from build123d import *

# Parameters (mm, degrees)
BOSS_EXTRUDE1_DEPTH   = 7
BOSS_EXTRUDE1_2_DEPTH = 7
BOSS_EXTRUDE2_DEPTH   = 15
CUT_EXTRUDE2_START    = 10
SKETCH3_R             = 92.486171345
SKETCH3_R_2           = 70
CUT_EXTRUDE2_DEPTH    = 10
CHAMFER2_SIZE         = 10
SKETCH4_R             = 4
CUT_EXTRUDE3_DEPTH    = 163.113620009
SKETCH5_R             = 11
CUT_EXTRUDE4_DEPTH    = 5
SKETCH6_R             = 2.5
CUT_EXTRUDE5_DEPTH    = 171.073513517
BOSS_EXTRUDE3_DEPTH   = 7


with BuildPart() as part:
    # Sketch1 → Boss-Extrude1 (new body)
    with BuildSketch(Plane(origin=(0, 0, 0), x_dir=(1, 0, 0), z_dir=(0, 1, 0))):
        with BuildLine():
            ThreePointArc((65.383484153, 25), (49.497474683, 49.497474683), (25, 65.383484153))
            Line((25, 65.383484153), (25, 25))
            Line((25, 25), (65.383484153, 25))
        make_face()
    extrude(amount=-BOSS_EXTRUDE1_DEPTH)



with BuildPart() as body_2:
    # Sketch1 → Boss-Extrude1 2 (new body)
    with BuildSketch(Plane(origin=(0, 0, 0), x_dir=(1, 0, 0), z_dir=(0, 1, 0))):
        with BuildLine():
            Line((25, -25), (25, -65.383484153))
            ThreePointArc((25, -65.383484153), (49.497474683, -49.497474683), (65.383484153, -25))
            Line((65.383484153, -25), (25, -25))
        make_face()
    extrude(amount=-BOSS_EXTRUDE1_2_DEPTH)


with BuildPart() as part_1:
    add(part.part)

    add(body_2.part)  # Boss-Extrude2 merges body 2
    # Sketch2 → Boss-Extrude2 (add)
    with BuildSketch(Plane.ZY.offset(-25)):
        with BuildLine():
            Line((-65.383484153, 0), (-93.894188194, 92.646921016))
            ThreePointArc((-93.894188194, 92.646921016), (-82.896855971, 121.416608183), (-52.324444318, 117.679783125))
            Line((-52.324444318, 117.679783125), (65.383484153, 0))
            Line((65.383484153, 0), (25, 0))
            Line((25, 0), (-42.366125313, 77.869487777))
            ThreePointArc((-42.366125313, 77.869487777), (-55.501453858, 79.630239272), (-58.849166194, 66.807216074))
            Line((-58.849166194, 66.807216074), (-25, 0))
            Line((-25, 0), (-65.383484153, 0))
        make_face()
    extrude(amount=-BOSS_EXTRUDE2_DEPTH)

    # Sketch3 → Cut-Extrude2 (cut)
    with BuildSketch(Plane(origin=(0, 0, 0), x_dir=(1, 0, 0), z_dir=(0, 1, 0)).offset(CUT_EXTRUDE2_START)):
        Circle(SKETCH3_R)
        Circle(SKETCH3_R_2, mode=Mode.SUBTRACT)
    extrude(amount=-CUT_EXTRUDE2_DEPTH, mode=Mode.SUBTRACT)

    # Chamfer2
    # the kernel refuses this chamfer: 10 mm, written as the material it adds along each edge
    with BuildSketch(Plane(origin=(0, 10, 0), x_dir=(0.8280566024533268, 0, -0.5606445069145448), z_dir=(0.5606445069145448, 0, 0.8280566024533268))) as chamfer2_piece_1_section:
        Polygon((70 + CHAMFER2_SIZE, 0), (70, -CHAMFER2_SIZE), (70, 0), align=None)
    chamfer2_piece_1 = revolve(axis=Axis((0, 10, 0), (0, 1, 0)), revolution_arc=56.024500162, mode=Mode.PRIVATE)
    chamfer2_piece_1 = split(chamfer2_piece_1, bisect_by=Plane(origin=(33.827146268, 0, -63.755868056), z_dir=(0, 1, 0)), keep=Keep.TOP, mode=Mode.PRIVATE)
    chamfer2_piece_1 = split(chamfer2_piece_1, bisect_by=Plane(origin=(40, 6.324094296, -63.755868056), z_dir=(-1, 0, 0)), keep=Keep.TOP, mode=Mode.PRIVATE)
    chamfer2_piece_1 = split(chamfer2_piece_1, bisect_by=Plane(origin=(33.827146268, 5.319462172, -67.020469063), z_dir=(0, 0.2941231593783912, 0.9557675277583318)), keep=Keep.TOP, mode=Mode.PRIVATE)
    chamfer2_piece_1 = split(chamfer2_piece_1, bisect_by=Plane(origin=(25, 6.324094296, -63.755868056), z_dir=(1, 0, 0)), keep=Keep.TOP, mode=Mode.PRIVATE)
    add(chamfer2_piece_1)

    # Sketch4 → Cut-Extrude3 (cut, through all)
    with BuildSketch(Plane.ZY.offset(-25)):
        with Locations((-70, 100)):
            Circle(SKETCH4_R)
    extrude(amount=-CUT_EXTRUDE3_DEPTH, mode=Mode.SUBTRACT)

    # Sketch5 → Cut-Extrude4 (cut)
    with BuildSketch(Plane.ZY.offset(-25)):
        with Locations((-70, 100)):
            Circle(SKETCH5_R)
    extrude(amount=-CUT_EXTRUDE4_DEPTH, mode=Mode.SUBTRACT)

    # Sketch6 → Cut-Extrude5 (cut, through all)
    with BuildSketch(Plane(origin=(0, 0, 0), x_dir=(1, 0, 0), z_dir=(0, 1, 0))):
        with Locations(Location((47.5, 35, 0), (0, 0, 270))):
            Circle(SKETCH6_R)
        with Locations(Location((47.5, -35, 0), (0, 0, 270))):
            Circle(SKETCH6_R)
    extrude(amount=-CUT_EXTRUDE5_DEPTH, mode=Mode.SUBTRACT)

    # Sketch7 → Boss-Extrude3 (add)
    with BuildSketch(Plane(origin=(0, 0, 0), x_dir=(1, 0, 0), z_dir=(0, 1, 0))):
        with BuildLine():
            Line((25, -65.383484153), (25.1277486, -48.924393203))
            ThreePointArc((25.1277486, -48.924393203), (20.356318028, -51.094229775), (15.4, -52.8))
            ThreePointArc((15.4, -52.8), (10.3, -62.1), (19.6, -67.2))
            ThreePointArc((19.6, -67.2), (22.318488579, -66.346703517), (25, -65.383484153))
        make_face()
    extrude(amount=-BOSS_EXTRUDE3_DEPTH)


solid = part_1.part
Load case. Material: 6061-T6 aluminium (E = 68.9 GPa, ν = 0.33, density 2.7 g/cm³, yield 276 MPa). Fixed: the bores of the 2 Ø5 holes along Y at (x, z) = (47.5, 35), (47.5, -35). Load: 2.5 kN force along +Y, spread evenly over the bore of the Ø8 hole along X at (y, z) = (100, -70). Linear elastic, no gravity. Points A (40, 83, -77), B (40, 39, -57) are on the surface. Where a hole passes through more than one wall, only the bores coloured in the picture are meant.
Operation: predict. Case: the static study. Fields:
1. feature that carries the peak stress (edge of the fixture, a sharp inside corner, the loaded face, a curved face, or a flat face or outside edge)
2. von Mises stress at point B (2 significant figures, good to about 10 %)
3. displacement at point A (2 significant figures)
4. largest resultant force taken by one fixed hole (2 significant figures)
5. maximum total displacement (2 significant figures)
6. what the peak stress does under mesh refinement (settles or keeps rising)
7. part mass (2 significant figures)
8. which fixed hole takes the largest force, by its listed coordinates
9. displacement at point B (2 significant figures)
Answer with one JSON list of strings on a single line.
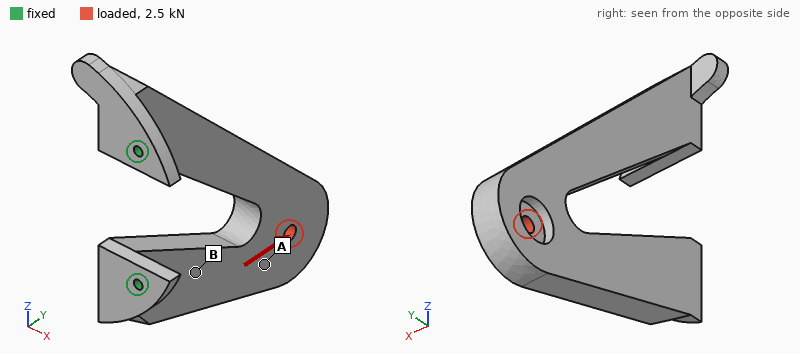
["edge of the fixture", "23 MPa", "0.34 mm", "3.5 kN", "0.43 mm", "keeps rising", "350 g", "(47.5, -35)", "0.20 mm"]
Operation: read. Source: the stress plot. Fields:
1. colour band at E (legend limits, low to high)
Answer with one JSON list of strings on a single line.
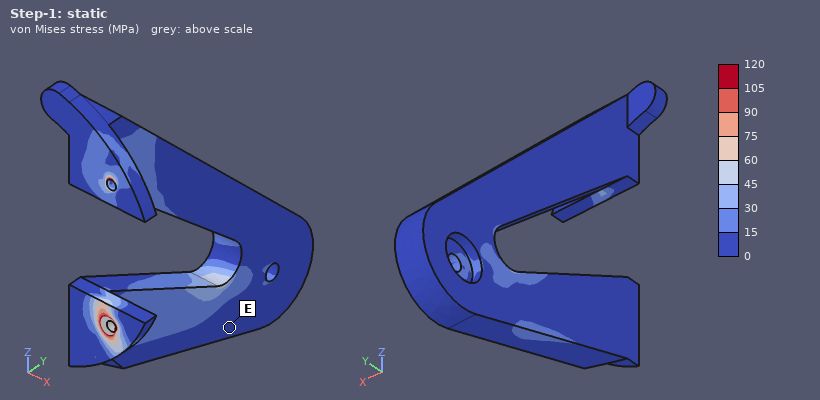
["0 to 15 MPa"]
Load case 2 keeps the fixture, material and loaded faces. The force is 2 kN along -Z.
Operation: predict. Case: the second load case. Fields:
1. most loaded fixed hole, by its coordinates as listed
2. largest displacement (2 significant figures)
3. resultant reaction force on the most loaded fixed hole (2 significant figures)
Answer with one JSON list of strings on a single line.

["(47.5, 35)", "0.32 mm", "3.3 kN"]
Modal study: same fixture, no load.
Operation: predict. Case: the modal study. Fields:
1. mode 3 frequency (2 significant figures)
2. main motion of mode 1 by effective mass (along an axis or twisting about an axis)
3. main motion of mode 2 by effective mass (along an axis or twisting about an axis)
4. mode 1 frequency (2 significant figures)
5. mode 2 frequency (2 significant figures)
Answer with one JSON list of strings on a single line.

["1600 Hz", "along X", "along Z", "330 Hz", "1000 Hz"]
